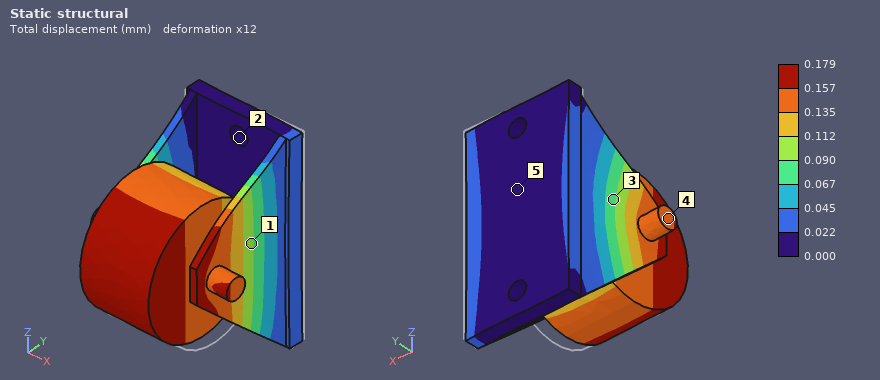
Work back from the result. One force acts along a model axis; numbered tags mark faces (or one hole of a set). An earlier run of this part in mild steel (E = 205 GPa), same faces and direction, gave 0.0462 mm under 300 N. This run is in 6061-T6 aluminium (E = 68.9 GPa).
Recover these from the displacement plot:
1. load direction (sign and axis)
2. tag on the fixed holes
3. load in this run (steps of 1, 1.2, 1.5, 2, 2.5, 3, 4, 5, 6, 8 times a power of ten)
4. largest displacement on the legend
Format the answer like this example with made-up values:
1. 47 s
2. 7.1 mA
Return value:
1. -X
2. 2
3. 400 N
4. 0.179 mm
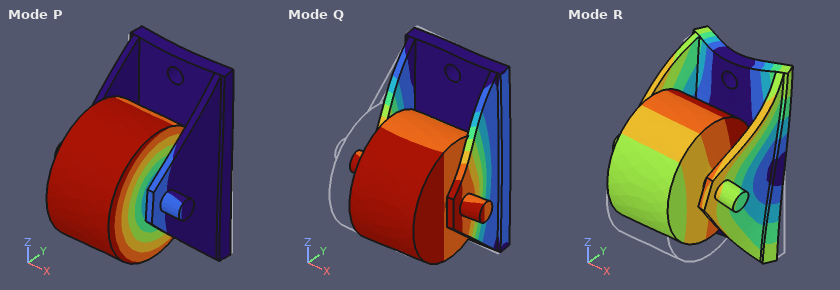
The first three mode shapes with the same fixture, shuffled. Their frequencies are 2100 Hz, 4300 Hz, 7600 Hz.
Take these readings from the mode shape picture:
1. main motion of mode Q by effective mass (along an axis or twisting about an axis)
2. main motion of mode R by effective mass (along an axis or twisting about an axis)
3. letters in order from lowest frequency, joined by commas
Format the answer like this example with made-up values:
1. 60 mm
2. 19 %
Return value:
1. along X
2. along Z
3. Q, P, R
